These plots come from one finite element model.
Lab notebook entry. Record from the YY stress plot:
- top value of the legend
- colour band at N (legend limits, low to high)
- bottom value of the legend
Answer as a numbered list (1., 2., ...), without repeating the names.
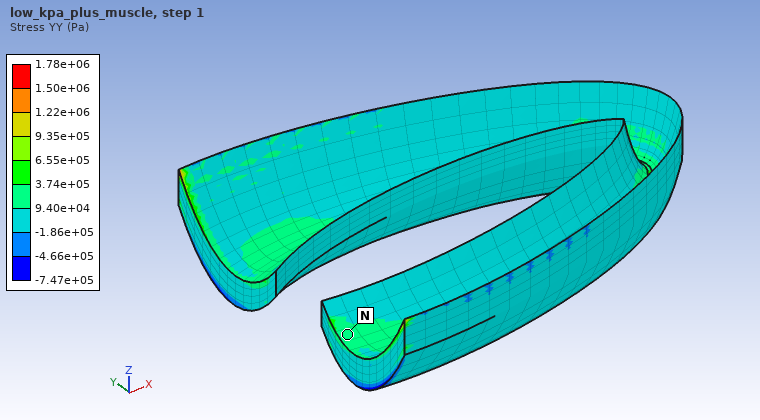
1. 1.78e+06 Pa
2. 9.40e+04 to 3.74e+05 Pa
3. -7.47e+05 Pa
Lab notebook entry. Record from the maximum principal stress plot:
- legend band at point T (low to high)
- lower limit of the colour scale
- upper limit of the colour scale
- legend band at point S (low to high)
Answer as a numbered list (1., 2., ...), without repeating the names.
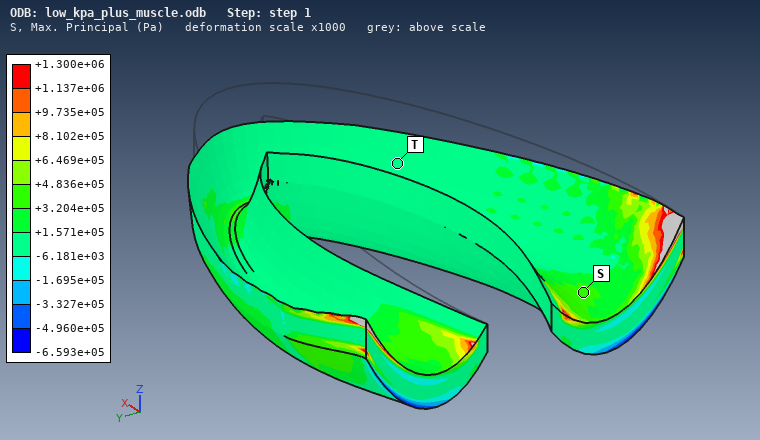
1. -6.181e+03 to +1.571e+05 Pa
2. -6.593e+05 Pa
3. +1.300e+06 Pa
4. +3.204e+05 to +4.836e+05 Pa
